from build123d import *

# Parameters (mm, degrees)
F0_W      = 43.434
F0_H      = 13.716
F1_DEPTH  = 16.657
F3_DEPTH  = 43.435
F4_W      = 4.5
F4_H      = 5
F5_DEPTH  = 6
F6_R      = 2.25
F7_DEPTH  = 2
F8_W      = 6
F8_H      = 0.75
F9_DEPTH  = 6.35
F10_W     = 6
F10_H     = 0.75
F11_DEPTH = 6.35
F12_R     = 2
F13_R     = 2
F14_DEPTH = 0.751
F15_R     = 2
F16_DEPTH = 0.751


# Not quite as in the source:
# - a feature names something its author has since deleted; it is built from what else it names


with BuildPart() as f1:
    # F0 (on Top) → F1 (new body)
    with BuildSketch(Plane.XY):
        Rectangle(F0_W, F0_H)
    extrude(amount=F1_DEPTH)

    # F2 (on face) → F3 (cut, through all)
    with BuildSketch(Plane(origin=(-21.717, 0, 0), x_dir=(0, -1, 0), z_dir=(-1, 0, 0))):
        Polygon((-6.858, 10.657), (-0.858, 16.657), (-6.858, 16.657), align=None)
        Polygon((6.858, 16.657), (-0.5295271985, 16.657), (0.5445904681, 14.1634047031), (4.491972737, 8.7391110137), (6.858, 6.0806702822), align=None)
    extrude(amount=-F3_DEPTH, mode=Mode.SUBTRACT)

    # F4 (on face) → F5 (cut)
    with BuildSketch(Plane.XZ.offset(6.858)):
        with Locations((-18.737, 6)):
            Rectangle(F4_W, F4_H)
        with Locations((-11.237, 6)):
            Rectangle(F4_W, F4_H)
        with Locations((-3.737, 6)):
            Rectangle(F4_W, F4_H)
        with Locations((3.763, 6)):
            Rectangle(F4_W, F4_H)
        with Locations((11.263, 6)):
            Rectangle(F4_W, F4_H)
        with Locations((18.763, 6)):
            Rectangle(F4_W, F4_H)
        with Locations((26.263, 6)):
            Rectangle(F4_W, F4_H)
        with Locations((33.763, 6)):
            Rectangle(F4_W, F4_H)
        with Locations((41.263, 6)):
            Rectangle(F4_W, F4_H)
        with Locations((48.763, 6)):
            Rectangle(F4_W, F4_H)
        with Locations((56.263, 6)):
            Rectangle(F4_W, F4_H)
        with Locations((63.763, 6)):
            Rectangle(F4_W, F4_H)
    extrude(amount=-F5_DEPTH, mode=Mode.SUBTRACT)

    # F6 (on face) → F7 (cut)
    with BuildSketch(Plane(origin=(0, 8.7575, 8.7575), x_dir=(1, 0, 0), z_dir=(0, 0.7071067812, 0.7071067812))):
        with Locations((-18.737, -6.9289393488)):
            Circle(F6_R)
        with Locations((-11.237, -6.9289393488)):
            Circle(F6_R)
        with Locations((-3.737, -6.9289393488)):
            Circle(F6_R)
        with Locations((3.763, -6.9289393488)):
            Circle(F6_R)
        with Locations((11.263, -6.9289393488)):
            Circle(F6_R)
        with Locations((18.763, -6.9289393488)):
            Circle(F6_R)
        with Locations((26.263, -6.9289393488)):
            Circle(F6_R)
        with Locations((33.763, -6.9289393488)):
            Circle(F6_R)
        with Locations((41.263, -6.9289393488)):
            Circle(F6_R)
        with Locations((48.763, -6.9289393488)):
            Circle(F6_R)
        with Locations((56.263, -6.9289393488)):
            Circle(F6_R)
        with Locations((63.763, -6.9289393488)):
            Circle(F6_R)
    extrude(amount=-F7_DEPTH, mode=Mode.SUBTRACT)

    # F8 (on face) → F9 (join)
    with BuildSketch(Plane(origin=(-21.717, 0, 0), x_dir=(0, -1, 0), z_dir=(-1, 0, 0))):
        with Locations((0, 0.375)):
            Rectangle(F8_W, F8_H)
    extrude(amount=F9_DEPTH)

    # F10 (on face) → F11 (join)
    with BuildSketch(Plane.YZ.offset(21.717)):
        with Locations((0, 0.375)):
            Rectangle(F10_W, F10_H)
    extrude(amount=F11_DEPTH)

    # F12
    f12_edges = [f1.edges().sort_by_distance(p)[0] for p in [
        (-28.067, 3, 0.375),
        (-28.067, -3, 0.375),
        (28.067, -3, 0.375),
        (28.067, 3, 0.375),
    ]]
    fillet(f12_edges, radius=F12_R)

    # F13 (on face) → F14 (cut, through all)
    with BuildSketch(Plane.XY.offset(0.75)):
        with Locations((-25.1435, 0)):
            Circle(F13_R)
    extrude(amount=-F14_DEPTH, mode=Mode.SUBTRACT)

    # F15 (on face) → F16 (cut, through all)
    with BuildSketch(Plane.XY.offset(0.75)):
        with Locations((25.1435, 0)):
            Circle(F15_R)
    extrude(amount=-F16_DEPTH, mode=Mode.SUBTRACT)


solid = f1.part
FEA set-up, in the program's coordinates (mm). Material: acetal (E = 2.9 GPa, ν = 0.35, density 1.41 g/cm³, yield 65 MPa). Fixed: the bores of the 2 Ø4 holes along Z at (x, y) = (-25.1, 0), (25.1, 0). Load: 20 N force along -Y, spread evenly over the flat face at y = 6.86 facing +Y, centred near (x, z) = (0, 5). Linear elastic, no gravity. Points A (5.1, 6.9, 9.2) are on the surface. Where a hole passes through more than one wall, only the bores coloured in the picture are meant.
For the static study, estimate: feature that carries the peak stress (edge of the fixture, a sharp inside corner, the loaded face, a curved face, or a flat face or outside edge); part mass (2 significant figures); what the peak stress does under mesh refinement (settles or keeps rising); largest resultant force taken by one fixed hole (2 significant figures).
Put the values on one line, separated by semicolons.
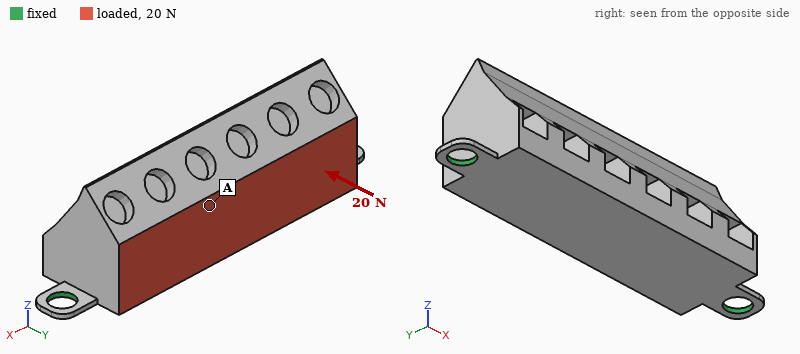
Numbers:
edge of the fixture; 8.9 g; keeps rising; 10 N
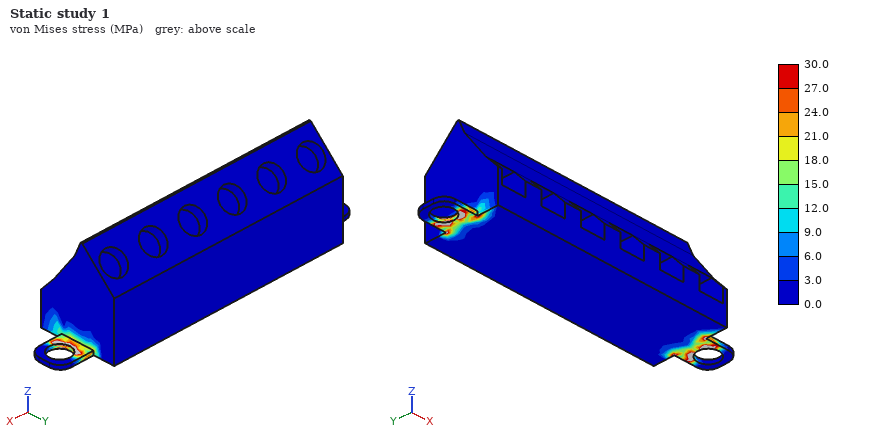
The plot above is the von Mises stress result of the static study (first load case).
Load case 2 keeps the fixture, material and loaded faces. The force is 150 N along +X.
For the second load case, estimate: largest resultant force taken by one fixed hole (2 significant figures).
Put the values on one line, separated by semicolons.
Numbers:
80 N
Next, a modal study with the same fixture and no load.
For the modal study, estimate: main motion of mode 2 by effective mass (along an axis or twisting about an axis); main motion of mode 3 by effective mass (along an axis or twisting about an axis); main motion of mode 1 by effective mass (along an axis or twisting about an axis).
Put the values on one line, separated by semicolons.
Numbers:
along Z; along X; along Y
